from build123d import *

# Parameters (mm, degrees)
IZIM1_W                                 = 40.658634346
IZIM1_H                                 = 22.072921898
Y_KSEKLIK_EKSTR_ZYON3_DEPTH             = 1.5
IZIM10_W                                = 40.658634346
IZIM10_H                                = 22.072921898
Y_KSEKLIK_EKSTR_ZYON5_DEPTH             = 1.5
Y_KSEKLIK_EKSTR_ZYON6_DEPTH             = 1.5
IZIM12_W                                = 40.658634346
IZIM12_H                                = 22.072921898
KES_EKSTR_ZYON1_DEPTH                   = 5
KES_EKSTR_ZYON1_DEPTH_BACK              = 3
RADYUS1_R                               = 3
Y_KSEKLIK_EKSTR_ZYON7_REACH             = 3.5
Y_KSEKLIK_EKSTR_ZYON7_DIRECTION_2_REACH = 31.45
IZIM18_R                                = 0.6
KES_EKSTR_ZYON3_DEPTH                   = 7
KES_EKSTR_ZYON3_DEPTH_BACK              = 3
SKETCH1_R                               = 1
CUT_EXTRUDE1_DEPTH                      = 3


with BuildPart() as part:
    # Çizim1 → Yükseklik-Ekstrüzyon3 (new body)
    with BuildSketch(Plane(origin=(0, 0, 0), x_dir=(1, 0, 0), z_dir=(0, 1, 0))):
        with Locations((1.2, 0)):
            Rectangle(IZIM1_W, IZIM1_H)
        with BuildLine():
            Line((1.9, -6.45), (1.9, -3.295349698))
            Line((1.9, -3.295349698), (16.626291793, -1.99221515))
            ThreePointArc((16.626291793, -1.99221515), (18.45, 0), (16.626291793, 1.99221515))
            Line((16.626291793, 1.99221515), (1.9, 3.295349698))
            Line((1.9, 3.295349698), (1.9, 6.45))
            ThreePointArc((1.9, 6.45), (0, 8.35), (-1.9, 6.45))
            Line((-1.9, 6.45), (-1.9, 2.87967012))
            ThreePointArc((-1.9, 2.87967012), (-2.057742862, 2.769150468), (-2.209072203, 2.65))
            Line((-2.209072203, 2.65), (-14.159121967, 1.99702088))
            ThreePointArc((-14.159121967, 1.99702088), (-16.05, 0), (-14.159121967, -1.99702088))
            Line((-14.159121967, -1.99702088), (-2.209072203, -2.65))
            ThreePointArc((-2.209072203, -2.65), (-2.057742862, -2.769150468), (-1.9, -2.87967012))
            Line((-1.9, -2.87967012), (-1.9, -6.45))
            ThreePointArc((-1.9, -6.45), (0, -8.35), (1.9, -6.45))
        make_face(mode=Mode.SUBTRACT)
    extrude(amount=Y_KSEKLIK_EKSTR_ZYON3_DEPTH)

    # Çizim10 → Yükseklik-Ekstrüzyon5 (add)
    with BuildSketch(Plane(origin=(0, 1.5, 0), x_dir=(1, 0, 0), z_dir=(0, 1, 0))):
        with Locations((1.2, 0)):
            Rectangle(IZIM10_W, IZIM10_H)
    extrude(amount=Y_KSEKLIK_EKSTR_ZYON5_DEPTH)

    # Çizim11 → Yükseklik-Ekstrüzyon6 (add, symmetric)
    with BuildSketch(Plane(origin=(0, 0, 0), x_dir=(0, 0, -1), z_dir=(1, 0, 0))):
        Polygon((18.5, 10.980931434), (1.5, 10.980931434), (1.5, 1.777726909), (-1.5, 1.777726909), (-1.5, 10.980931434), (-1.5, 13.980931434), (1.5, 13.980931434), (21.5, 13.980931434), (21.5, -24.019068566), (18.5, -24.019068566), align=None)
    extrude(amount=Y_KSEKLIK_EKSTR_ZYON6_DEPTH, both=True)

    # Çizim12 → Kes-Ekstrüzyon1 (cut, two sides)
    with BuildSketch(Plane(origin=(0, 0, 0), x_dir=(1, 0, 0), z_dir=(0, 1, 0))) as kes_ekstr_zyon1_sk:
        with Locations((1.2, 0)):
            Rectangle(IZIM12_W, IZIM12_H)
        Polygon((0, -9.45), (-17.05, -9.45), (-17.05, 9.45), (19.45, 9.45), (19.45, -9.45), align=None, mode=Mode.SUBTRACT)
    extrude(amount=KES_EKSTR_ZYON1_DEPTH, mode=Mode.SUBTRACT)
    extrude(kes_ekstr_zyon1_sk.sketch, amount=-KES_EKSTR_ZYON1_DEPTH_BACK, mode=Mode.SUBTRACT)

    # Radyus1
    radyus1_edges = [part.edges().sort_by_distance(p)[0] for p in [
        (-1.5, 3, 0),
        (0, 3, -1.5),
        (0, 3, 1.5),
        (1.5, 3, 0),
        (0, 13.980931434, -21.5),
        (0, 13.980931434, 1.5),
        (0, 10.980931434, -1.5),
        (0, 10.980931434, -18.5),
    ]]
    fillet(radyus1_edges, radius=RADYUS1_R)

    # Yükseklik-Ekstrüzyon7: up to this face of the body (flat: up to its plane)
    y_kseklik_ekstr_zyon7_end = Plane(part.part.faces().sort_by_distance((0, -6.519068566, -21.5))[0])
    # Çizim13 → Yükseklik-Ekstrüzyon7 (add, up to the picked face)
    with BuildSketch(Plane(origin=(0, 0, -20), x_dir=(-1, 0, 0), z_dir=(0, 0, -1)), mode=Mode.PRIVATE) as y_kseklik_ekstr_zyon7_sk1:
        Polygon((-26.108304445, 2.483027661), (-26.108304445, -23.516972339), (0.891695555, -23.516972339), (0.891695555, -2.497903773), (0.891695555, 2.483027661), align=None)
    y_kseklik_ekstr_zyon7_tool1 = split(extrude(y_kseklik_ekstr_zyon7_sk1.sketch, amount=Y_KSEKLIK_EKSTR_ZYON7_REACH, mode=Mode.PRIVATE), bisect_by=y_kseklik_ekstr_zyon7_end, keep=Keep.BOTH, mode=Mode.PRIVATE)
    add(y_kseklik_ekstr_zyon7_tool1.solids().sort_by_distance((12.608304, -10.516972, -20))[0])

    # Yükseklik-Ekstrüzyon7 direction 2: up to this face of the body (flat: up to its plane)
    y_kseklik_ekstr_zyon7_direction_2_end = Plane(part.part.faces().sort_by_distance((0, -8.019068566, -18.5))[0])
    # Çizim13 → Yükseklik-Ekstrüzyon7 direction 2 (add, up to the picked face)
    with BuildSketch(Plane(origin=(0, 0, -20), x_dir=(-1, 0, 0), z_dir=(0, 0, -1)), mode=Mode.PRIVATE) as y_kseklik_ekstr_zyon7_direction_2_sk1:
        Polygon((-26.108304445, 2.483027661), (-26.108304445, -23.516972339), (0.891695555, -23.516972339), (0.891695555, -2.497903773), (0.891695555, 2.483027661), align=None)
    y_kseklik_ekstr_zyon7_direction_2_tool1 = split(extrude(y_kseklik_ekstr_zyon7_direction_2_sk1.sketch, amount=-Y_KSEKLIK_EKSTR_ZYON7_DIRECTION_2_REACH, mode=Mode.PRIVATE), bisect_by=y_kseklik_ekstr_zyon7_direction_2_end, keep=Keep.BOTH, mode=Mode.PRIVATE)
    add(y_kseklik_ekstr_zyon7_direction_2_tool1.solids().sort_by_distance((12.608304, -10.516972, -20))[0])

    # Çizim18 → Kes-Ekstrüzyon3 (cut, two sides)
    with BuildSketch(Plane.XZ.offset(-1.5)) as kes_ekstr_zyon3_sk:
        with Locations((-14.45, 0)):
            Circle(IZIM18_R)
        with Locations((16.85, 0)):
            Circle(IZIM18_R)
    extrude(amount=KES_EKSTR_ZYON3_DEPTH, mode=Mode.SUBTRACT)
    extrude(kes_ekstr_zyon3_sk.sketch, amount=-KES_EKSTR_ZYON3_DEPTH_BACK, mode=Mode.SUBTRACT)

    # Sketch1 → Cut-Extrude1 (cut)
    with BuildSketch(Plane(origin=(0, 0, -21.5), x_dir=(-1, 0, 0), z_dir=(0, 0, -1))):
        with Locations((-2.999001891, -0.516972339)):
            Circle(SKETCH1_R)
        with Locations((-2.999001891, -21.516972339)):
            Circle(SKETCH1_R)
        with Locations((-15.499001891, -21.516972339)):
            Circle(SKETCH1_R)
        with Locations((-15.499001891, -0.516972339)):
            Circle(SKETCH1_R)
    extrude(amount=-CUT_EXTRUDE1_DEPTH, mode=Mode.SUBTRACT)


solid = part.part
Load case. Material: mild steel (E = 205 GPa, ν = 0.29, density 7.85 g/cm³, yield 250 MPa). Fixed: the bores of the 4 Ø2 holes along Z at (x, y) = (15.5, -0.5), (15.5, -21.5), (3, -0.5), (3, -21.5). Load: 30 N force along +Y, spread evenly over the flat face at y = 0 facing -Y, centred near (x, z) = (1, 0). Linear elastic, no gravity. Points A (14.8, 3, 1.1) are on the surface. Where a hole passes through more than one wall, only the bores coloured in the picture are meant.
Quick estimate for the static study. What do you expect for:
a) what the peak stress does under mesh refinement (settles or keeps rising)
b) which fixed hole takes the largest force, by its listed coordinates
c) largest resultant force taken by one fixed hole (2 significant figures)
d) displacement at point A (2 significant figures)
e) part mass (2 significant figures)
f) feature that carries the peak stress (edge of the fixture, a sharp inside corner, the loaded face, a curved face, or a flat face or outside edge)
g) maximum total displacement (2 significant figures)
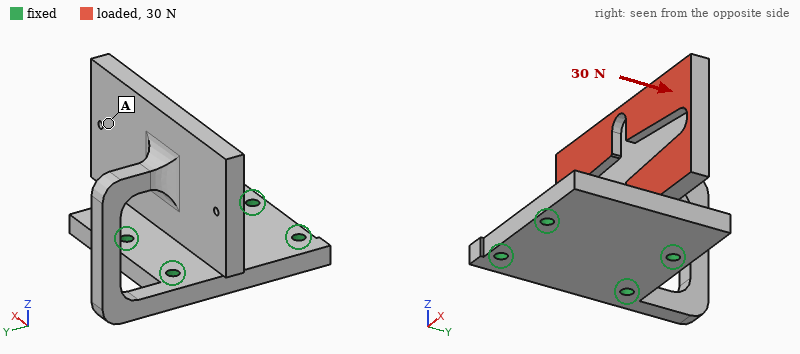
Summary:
keeps rising
(3, -0.5)
28 N
0.17 mm
33 g
a sharp inside corner
0.25 mm
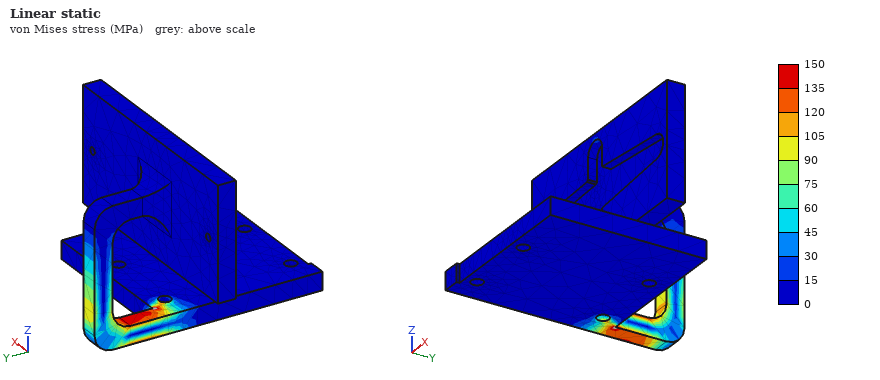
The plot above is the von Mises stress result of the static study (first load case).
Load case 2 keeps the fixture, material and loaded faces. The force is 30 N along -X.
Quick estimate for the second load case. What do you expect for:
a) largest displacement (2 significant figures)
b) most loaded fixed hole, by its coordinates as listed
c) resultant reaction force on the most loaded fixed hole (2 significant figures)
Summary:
0.46 mm
(3, -0.5)
29 N
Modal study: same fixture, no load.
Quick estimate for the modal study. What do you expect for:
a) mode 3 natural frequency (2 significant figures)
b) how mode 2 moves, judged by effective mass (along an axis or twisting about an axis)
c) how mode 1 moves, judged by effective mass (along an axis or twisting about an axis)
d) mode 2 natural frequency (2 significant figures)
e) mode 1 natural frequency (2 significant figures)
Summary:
680 Hz
along Y
along X
530 Hz
390 Hz
